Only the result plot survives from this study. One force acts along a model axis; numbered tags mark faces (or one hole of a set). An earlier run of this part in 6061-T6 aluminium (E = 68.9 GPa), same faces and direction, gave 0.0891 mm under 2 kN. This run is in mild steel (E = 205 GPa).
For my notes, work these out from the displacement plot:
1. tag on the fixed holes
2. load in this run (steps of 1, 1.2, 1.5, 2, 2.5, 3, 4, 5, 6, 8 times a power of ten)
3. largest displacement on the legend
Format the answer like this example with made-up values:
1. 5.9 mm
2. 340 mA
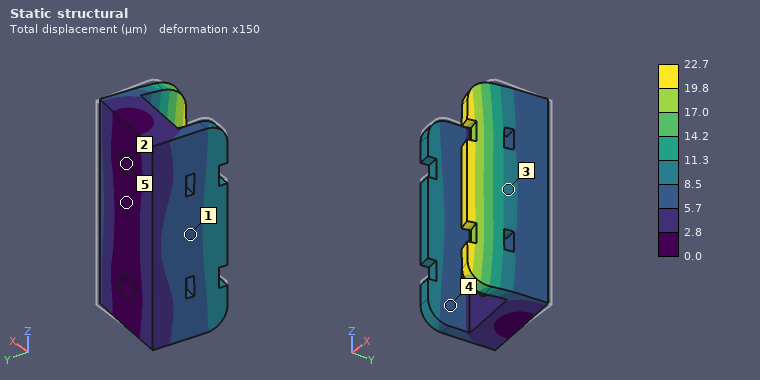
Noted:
1. 2
2. 1.5 kN
3. 22.7 µm
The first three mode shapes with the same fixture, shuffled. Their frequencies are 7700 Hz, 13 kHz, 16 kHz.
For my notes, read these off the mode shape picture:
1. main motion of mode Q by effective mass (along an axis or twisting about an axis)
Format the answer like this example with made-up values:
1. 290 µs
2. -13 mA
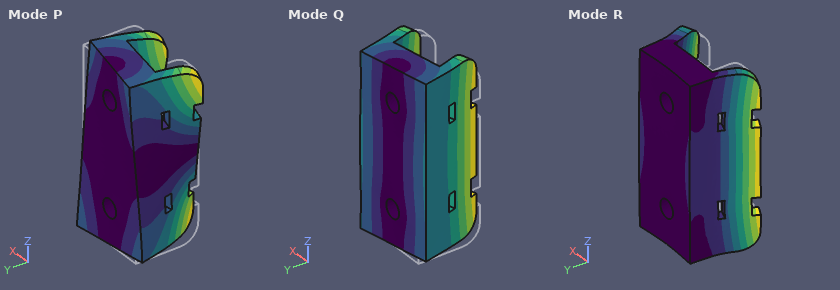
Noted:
1. along X
